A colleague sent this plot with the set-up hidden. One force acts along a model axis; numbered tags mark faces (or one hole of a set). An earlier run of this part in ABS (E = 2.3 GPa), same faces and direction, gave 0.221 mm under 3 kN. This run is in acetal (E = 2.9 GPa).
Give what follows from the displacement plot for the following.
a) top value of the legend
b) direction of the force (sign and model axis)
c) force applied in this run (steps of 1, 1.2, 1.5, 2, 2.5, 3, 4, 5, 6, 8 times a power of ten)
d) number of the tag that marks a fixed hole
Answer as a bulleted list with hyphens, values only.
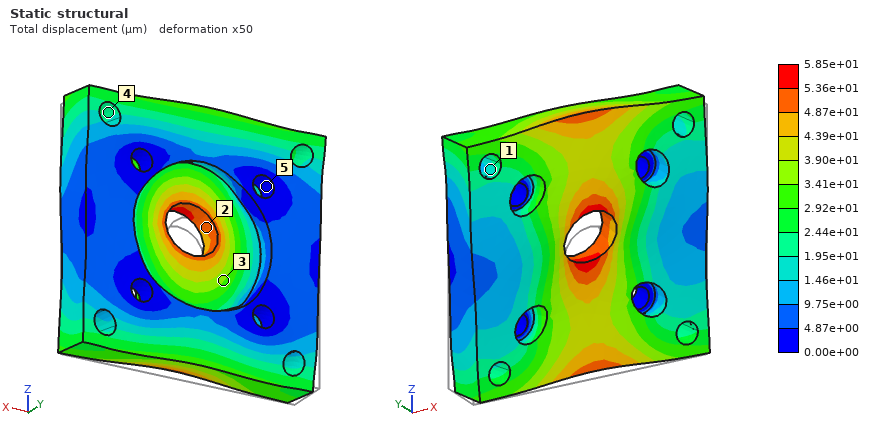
- 5.85e+01 µm
- +Z
- 1 kN
- 5
